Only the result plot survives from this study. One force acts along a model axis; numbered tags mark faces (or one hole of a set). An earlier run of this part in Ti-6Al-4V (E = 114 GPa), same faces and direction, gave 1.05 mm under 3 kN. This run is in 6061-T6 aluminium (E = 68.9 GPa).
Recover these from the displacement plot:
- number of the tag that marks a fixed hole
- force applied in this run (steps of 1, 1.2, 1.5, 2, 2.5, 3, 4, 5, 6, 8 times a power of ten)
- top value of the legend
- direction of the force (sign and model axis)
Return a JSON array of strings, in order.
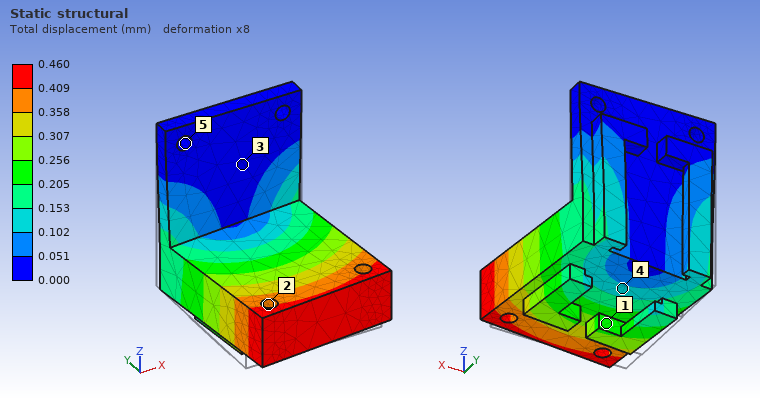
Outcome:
["5", "800 N", "0.460 mm", "+X"]
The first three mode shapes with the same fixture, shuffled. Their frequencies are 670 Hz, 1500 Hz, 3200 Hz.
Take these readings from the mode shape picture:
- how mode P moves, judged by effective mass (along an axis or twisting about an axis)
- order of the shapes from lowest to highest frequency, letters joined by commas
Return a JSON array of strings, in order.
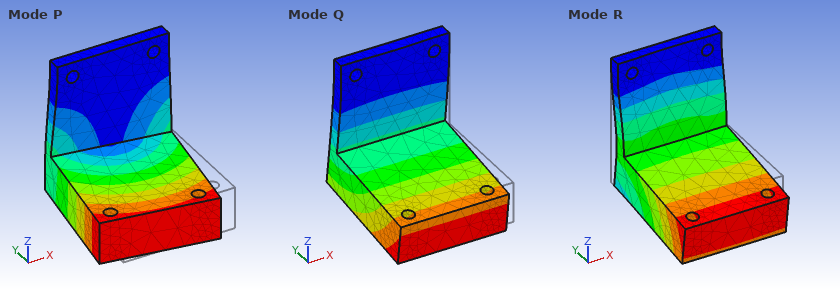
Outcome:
["along X", "Q, P, R"]
